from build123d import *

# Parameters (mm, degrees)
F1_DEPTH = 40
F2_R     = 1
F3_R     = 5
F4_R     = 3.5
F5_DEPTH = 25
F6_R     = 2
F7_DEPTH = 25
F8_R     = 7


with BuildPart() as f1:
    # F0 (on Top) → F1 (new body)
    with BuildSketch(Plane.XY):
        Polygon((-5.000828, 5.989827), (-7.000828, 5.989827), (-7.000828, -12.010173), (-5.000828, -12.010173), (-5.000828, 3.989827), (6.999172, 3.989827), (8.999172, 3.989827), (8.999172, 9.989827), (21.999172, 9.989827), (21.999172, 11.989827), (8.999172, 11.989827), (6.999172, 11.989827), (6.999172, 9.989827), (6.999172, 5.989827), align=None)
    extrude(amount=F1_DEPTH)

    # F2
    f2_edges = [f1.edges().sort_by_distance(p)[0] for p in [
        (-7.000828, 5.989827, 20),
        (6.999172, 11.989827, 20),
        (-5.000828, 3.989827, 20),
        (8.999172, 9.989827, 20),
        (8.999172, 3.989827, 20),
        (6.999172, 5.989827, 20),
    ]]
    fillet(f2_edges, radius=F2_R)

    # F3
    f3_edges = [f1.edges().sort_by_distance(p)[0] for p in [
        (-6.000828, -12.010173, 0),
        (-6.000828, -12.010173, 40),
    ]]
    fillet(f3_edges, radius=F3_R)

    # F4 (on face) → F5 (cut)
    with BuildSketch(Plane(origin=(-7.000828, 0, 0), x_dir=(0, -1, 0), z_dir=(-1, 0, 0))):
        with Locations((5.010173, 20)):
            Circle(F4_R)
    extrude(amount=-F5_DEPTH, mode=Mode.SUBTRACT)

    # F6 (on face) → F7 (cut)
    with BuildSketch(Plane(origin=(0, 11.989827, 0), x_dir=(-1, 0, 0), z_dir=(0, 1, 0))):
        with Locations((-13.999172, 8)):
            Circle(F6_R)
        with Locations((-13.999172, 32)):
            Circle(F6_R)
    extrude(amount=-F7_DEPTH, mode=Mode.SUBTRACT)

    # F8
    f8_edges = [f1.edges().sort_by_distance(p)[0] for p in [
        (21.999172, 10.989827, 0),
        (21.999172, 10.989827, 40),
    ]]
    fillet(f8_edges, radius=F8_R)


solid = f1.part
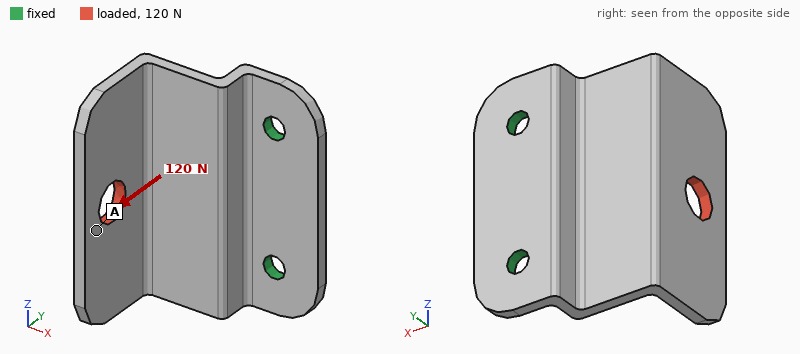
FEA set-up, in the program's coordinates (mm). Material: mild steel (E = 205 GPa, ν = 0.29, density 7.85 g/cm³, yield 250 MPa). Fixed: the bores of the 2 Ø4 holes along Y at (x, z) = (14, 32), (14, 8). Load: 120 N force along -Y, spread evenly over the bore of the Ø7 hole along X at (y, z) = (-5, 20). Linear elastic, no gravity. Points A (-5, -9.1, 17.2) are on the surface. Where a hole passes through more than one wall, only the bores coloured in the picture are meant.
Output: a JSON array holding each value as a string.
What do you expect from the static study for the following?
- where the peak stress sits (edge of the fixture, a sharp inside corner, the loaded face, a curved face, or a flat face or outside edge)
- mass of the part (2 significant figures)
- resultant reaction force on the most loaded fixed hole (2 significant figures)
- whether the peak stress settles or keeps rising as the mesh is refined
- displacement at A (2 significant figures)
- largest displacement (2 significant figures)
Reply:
["edge of the fixture", "31 g", "65 N", "keeps rising", "0.10 mm", "0.12 mm"]
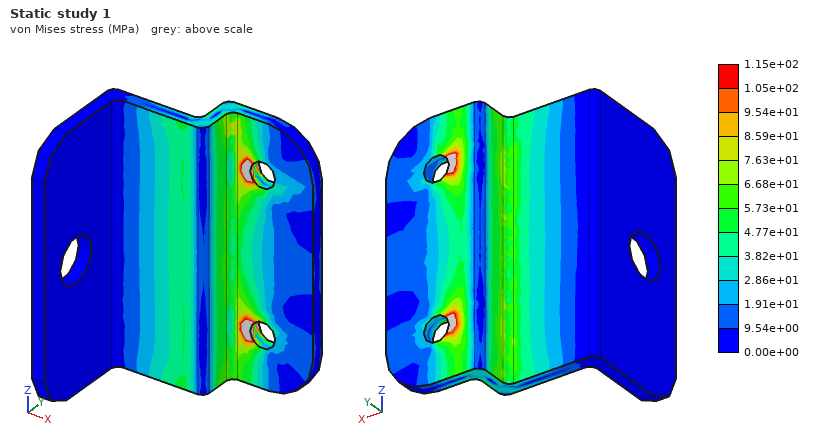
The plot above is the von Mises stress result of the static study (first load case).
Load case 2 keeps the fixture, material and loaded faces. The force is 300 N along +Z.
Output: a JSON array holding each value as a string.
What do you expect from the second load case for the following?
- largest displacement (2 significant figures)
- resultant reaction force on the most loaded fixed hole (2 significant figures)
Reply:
["51 µm", "330 N"]
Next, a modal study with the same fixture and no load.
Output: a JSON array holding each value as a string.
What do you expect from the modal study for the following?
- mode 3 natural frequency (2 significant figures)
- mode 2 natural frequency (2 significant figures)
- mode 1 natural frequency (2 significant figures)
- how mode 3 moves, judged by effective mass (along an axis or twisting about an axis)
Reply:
["5700 Hz", "3100 Hz", "1400 Hz", "along Y"]
